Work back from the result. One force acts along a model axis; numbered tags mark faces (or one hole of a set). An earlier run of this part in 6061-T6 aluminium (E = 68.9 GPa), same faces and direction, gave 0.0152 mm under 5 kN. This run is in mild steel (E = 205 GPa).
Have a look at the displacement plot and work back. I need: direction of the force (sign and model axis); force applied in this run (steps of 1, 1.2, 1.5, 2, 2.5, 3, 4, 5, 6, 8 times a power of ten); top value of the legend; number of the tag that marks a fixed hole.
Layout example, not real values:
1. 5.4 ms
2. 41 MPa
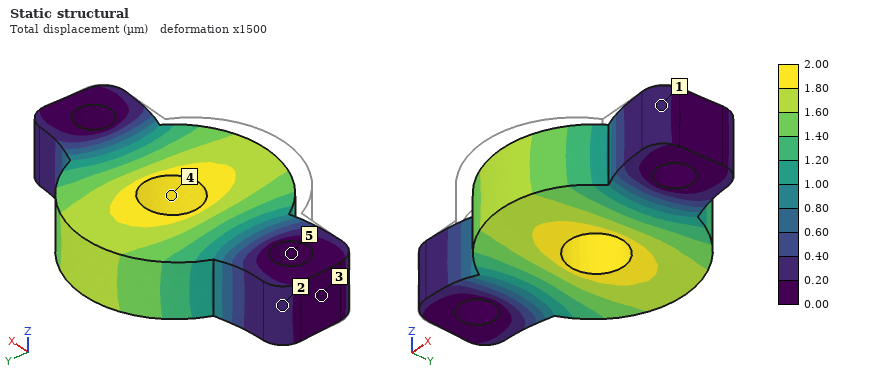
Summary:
1. +Y
2. 2 kN
3. 2.00 µm
4. 5
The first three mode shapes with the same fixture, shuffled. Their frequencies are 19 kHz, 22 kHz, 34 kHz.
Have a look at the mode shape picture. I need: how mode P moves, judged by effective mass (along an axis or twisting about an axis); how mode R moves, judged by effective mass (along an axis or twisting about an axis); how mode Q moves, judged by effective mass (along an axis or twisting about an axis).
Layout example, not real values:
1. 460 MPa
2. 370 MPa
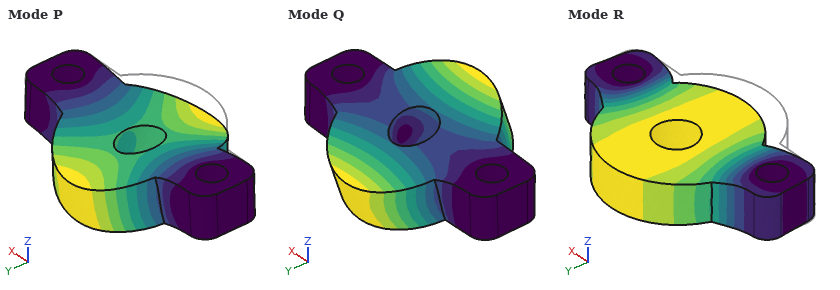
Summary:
1. along Z
2. along Y
3. twisting about X
